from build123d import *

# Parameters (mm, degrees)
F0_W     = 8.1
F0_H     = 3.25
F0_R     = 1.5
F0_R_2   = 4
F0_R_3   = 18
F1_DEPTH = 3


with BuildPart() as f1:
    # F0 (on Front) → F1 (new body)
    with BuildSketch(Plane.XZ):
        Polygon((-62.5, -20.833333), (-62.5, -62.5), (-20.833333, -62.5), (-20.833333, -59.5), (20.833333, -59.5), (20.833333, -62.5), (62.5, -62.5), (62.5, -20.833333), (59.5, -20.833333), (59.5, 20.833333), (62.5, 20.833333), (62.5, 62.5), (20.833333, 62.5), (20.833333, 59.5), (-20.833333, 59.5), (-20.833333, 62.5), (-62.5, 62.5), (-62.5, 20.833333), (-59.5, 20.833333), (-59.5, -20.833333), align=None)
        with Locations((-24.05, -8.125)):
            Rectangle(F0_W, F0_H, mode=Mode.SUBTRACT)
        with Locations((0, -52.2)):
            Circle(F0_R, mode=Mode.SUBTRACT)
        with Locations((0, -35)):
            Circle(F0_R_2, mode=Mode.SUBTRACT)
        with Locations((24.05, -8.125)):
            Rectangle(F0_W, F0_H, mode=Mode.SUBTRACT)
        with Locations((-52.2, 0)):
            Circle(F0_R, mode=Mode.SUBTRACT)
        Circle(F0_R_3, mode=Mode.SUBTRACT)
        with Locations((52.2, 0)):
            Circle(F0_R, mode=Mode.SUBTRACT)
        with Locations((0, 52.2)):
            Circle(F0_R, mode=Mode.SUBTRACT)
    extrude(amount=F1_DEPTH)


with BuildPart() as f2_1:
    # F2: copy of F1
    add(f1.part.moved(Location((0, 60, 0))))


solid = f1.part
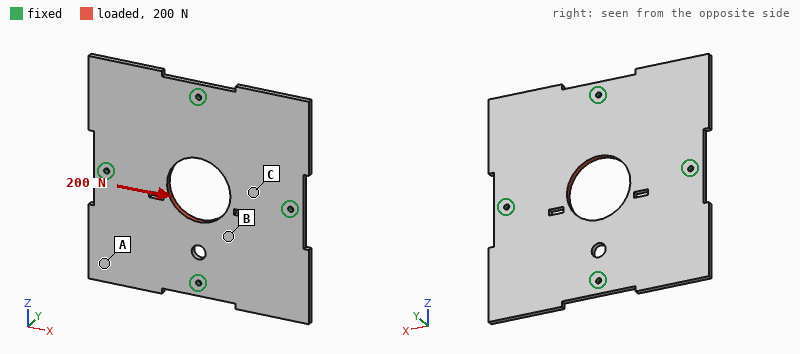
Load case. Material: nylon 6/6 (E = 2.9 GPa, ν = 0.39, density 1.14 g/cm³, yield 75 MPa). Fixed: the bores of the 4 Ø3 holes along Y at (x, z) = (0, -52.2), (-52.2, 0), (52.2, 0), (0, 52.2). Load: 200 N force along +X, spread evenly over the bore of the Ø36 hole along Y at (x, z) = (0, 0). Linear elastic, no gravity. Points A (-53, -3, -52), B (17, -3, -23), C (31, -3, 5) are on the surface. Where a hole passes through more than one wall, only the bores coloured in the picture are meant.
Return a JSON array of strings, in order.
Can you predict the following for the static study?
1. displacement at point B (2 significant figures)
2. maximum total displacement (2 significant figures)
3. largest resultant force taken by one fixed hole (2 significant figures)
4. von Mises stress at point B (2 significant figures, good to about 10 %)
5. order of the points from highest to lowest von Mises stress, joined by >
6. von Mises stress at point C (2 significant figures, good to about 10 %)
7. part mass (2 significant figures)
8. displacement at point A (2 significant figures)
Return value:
["9.8 µm", "13 µm", "58 N", "0.40 MPa", "C > B > A", "0.74 MPa", "48 g", "5.8 µm"]
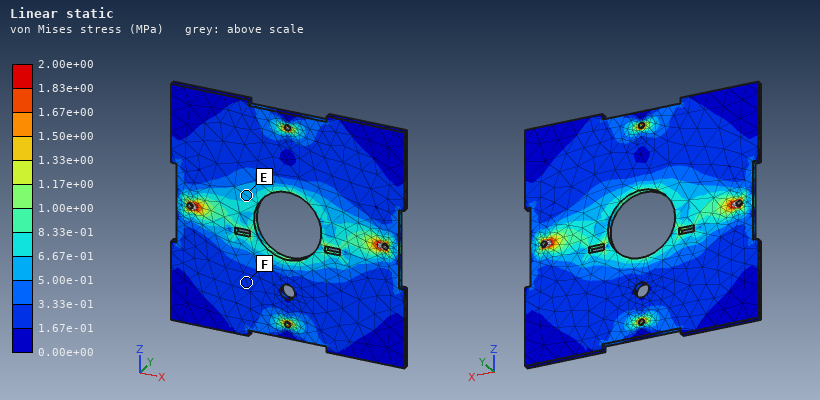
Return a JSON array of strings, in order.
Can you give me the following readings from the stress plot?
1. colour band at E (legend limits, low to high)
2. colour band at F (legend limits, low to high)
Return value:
["5.00e-01 to 6.67e-01 MPa", "1.67e-01 to 3.33e-01 MPa"]
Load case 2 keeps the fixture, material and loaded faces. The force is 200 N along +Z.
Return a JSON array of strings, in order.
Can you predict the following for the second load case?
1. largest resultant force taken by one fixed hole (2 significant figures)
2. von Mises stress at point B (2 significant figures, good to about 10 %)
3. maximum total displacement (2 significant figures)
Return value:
["60 N", "0.56 MPa", "14 µm"]
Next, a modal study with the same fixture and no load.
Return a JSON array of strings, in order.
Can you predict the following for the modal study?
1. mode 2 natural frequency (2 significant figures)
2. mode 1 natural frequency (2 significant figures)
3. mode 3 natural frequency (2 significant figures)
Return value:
["360 Hz", "340 Hz", "360 Hz"]
